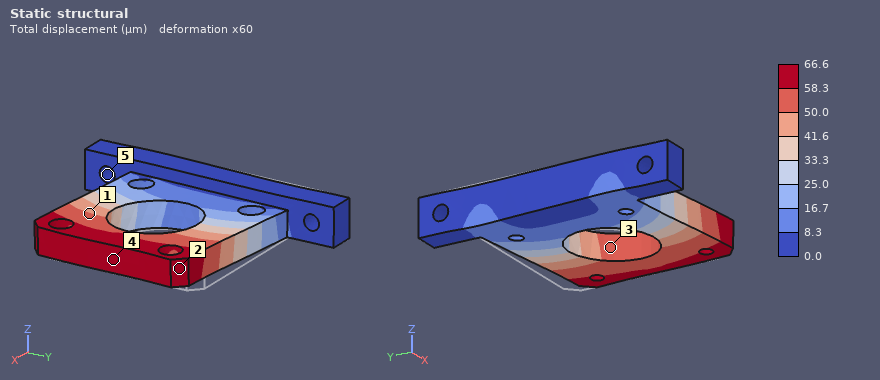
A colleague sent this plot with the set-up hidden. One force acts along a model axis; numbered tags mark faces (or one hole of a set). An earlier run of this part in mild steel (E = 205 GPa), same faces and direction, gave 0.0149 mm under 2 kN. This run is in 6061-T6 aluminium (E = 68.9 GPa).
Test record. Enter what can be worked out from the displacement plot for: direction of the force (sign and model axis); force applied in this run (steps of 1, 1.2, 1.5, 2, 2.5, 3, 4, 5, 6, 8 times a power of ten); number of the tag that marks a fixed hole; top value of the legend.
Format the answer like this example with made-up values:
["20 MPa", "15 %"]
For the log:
["-Y", "3 kN", "5", "66.6 µm"]
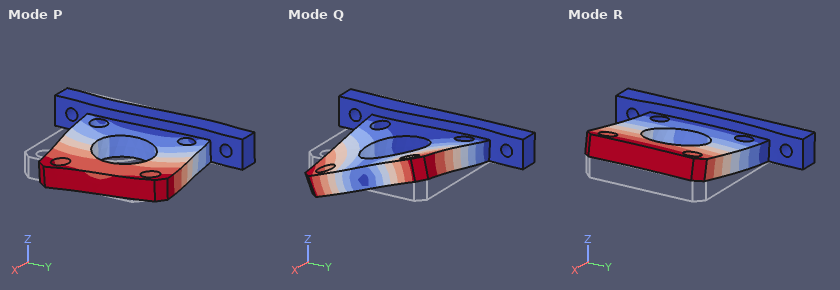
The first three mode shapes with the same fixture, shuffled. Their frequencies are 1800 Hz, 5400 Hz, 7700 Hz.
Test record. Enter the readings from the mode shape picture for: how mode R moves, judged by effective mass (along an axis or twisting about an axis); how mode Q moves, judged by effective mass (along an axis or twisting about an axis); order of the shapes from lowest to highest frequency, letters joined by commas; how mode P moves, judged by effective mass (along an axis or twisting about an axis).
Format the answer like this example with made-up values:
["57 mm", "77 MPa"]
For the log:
["along Z", "twisting about X", "R, Q, P", "along Y"]
